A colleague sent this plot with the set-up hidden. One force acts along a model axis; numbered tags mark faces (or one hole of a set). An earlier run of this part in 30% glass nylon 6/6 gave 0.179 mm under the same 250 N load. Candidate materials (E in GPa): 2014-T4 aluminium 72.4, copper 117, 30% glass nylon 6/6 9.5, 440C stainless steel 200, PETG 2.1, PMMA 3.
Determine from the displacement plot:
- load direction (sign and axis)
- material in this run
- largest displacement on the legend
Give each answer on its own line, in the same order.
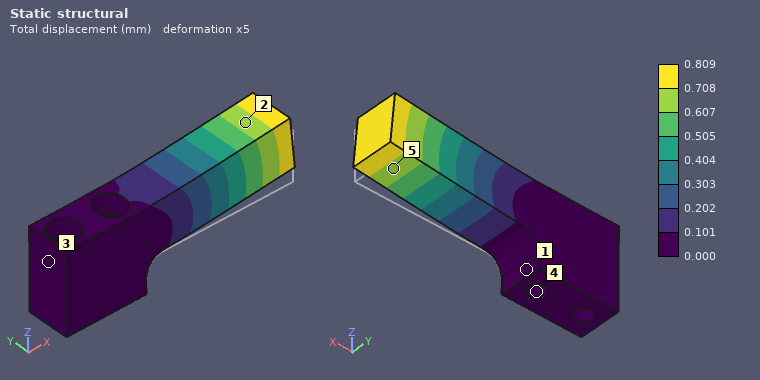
+Z
PETG
0.809 mm
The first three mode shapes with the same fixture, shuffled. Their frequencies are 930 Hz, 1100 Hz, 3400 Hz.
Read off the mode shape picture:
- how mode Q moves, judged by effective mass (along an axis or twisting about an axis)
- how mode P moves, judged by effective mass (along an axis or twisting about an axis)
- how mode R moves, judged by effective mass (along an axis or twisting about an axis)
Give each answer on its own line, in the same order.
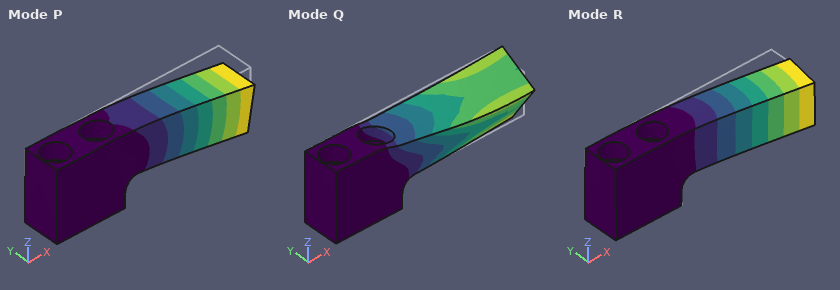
twisting about X
along Z
along Y
